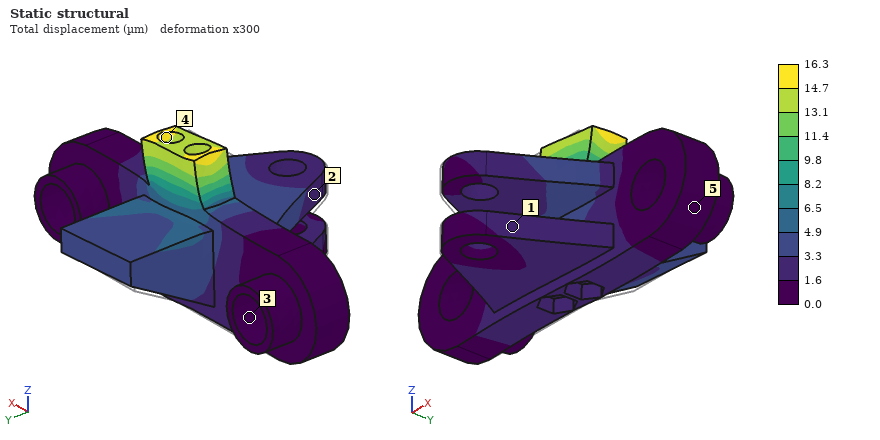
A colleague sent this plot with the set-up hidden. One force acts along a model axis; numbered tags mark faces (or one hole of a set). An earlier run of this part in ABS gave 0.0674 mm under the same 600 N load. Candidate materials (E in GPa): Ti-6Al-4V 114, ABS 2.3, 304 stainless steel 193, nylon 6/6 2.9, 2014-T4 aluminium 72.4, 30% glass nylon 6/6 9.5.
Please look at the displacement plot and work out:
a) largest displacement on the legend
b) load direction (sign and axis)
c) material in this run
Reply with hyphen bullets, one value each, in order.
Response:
- 16.3 µm
- +X
- 30% glass nylon 6/6
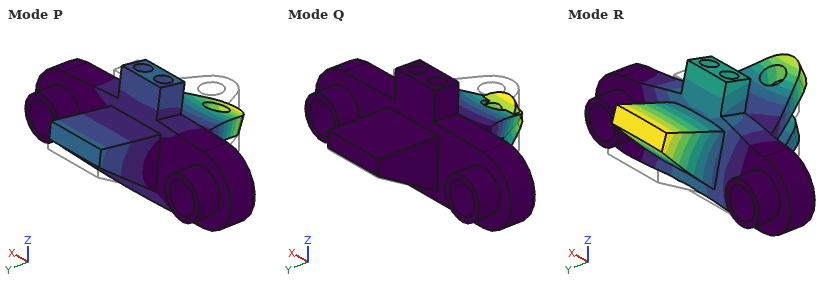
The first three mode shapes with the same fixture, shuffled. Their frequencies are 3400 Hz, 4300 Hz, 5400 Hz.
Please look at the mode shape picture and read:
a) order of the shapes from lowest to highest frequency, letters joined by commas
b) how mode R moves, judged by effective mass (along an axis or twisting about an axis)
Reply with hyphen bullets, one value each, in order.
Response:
- P, Q, R
- along Z
